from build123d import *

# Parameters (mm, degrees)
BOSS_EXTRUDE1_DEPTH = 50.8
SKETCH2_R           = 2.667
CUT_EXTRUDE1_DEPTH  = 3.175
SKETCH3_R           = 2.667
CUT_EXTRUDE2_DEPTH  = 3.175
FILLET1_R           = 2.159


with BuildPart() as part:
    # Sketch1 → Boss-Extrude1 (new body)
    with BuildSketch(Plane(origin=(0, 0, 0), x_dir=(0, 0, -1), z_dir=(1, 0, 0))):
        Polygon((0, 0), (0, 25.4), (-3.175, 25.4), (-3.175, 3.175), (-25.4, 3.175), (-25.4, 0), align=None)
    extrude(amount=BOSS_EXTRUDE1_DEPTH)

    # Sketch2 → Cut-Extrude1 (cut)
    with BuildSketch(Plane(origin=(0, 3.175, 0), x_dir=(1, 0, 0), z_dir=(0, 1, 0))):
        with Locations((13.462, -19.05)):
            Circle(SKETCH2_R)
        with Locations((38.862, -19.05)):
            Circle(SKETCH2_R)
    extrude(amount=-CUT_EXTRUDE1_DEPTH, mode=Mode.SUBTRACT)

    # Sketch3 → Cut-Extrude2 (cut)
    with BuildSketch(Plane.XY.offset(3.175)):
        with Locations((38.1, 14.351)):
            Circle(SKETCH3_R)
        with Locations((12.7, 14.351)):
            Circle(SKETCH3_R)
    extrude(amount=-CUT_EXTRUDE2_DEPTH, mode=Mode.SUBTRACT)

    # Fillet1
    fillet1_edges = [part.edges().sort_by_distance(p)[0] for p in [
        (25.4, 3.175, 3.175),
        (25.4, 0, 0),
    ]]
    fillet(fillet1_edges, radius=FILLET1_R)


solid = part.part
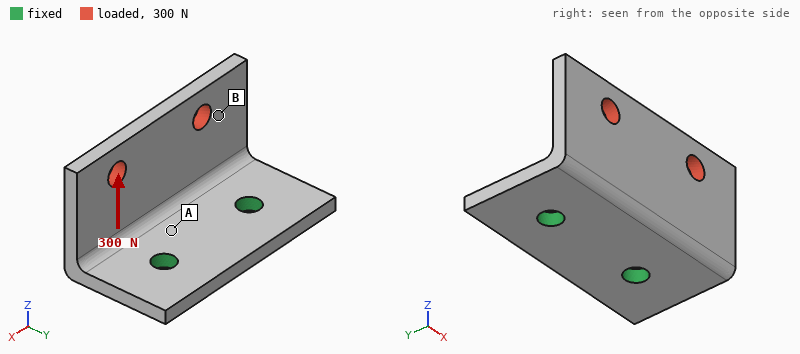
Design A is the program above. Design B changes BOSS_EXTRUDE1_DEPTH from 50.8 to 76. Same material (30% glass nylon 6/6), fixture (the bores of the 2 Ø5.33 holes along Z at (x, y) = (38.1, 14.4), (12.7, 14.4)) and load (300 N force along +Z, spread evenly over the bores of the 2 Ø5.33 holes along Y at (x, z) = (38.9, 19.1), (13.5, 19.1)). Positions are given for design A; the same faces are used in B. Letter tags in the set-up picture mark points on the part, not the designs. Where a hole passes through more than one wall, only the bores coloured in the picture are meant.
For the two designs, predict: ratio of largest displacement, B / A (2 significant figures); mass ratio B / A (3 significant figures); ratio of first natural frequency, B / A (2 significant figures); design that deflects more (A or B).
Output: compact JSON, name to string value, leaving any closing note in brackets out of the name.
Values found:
{"ratio of largest displacement, B / A": "0.91", "mass ratio B / A": "1.52", "ratio of first natural frequency, B / A": "0.79", "design that deflects more": "A"}
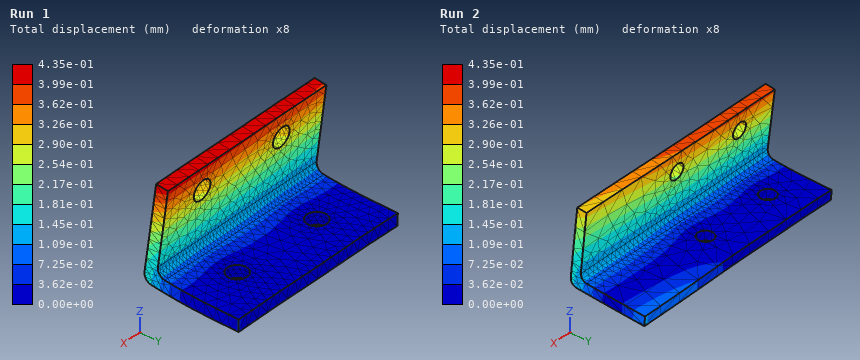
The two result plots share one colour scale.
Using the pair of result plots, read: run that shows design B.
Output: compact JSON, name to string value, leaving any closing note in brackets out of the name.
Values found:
{"run that shows design B": "Run 2"}
